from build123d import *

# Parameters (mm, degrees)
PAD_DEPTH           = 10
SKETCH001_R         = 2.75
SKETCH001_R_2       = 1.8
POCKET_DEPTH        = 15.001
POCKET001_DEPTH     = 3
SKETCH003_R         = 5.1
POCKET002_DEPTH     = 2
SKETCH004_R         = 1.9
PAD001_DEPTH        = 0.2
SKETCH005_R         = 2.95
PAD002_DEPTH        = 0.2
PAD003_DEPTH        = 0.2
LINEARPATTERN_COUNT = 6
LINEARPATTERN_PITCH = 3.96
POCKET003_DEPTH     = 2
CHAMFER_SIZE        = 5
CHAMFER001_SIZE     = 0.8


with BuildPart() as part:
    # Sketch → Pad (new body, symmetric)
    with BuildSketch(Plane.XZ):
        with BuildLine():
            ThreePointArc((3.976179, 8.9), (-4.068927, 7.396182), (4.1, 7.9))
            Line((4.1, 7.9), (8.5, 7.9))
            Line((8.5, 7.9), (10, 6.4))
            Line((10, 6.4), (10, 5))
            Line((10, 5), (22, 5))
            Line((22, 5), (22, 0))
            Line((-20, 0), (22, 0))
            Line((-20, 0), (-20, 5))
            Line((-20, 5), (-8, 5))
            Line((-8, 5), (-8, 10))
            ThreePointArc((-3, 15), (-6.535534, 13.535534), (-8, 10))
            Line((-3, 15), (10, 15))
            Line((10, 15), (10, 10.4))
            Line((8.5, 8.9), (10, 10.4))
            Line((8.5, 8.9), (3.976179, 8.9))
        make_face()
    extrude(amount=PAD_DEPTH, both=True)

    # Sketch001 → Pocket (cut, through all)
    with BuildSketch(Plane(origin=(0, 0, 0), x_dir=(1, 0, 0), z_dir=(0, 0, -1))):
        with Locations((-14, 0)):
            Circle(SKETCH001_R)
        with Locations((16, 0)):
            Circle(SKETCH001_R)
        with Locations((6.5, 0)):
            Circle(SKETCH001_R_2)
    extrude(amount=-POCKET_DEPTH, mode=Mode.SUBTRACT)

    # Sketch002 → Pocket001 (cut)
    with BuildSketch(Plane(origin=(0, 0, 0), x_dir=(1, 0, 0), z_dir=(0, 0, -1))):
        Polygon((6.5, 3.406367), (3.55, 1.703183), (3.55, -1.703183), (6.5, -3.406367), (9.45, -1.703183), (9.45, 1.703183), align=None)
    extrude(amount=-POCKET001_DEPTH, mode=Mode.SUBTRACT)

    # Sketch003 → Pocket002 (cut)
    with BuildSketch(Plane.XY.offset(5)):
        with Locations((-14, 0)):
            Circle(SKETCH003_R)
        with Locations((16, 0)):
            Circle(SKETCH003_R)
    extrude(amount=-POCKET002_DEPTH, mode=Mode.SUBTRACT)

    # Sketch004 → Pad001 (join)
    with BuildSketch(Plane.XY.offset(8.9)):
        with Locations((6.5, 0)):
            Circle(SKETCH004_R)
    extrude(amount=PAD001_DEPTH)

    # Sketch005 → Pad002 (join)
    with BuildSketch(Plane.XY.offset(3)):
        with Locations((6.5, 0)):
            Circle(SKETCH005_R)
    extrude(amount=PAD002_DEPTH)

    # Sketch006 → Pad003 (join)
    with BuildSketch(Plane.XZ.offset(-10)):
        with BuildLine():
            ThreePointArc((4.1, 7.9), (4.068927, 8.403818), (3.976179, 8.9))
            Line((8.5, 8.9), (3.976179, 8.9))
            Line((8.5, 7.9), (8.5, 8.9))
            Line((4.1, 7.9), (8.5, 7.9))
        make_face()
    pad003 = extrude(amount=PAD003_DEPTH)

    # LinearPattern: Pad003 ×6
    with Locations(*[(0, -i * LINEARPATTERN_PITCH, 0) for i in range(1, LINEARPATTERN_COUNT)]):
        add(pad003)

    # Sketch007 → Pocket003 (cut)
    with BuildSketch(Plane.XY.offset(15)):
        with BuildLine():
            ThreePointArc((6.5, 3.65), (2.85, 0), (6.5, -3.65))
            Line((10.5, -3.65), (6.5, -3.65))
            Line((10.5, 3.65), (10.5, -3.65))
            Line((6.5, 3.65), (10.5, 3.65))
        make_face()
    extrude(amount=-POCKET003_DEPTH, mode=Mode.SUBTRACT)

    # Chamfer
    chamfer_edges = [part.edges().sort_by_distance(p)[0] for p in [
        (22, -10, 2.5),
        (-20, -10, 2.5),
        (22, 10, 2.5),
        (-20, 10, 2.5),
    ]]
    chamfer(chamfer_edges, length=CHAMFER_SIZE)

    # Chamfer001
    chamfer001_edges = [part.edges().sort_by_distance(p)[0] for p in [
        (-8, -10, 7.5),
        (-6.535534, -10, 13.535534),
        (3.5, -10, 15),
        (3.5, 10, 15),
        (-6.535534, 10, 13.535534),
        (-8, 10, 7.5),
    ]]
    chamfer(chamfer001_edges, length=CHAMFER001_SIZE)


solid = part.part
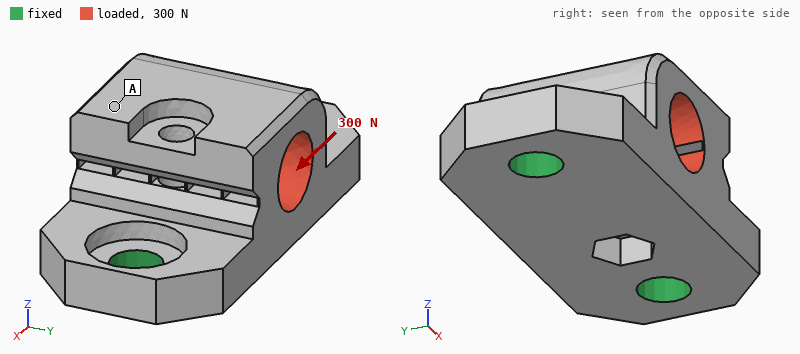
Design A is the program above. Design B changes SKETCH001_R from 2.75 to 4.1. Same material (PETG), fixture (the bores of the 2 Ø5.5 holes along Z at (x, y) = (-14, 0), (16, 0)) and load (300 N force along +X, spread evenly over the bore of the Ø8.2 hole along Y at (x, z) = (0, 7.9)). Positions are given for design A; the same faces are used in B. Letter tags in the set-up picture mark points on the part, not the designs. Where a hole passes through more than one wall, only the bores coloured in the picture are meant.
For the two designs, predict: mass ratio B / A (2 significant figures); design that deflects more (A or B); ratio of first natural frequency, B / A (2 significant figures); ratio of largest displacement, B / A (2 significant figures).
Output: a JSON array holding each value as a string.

["0.97", "A", "1.3", "0.83"]
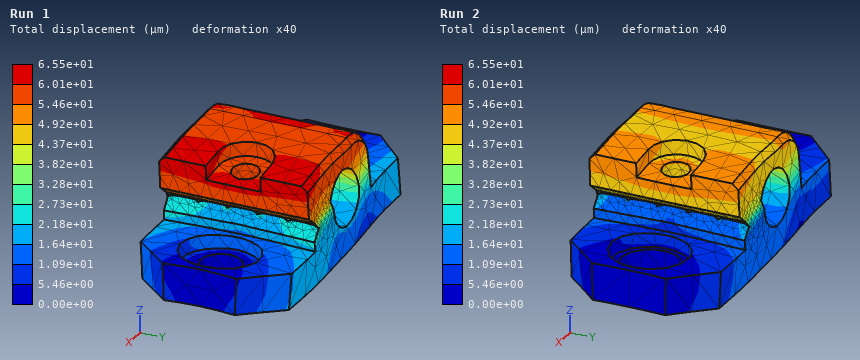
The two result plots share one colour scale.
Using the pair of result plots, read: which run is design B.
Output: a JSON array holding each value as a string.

["Run 2"]
